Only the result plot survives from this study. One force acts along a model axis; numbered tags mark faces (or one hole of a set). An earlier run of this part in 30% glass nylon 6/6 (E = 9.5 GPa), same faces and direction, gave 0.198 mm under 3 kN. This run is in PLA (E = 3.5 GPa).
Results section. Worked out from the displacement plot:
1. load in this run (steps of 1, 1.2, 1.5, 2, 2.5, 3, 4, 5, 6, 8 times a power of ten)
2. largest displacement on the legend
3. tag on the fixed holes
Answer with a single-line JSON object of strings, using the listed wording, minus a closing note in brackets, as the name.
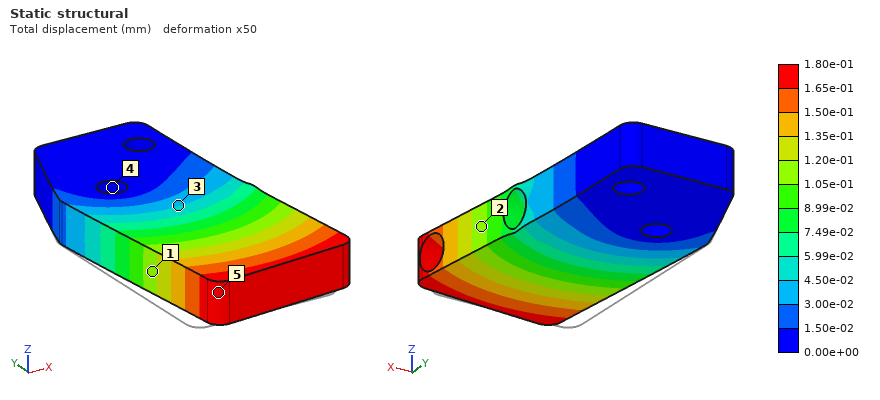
{"load in this run": "1 kN", "largest displacement on the legend": "1.80e-01 mm", "tag on the fixed holes": "4"}
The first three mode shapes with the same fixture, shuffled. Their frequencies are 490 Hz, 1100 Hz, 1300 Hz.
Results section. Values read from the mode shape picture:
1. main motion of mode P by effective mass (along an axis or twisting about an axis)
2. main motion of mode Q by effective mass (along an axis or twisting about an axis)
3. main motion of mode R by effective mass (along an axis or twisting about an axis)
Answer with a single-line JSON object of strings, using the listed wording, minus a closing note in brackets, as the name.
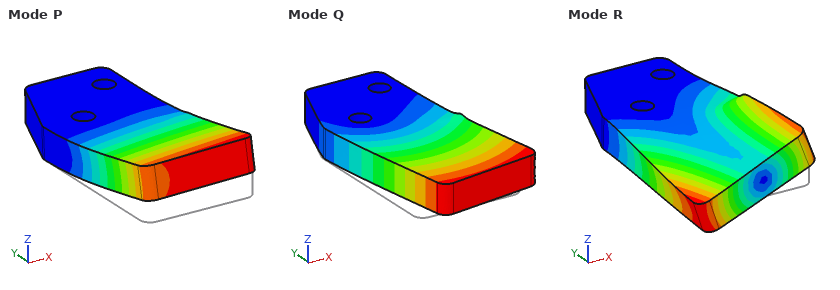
{"main motion of mode P by effective mass": "along Z", "main motion of mode Q by effective mass": "along X", "main motion of mode R by effective mass": "twisting about Y"}
